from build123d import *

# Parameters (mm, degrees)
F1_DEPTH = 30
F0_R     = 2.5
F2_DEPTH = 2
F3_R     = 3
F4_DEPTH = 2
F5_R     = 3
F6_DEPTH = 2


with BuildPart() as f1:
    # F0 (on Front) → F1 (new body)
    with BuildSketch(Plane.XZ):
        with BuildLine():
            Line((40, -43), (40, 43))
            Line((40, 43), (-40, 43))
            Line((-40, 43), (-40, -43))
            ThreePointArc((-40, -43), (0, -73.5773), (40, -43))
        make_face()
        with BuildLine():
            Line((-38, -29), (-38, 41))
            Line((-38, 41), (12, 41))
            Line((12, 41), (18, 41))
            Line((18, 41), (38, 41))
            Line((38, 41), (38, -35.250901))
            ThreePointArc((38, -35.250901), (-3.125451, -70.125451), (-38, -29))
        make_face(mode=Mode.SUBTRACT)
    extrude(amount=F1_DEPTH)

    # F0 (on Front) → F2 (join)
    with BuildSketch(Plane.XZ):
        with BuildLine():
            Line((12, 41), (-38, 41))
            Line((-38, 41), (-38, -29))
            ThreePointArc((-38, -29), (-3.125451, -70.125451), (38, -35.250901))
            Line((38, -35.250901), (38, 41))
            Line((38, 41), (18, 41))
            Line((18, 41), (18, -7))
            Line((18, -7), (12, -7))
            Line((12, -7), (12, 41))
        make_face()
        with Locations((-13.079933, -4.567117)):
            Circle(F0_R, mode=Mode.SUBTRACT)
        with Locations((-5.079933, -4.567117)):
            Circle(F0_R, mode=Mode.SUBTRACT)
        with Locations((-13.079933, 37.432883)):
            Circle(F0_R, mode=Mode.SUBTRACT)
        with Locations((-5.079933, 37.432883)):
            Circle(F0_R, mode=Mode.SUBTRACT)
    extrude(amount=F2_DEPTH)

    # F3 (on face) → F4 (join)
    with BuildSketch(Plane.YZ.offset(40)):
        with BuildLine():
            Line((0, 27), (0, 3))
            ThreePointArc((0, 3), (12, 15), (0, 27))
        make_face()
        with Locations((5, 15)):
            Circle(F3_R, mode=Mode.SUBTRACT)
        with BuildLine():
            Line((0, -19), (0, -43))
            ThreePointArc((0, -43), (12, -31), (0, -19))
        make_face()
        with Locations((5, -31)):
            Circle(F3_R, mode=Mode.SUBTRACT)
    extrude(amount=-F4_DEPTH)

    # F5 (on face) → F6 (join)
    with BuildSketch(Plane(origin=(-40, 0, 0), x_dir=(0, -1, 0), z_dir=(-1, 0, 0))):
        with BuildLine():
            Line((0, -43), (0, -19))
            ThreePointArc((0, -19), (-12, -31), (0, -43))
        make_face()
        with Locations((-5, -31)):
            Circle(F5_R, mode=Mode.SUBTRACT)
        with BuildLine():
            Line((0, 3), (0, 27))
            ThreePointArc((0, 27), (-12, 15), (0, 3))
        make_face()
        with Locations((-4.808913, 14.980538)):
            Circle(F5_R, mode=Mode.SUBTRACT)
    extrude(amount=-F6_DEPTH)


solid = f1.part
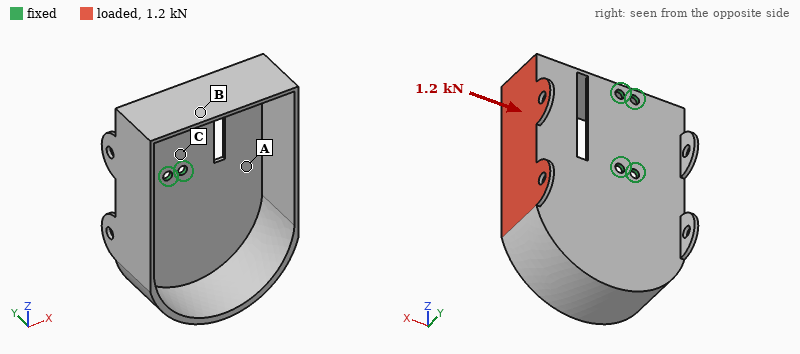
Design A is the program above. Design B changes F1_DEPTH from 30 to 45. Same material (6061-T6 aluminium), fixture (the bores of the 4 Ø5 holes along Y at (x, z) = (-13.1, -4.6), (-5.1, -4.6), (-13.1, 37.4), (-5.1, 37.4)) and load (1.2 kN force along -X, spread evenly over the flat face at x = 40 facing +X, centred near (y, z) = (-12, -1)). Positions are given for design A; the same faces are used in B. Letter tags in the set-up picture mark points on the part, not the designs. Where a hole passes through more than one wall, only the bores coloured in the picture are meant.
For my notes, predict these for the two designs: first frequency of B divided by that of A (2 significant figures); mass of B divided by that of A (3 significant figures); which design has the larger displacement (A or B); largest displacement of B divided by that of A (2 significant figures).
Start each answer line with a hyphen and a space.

- 0.87
- 1.30
- B
- 1.5
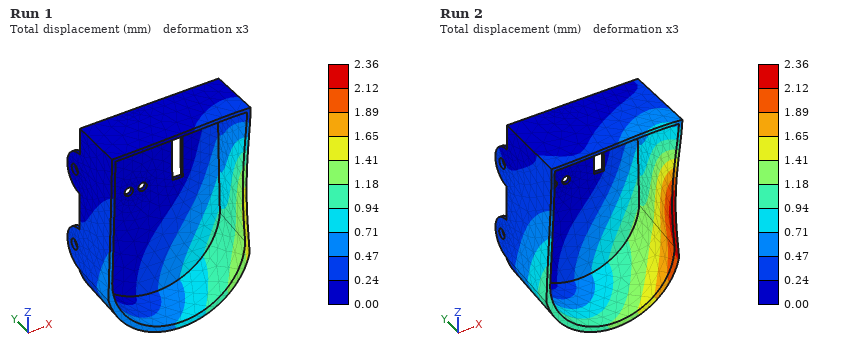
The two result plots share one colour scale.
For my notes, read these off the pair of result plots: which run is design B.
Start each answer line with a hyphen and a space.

- Run 2
